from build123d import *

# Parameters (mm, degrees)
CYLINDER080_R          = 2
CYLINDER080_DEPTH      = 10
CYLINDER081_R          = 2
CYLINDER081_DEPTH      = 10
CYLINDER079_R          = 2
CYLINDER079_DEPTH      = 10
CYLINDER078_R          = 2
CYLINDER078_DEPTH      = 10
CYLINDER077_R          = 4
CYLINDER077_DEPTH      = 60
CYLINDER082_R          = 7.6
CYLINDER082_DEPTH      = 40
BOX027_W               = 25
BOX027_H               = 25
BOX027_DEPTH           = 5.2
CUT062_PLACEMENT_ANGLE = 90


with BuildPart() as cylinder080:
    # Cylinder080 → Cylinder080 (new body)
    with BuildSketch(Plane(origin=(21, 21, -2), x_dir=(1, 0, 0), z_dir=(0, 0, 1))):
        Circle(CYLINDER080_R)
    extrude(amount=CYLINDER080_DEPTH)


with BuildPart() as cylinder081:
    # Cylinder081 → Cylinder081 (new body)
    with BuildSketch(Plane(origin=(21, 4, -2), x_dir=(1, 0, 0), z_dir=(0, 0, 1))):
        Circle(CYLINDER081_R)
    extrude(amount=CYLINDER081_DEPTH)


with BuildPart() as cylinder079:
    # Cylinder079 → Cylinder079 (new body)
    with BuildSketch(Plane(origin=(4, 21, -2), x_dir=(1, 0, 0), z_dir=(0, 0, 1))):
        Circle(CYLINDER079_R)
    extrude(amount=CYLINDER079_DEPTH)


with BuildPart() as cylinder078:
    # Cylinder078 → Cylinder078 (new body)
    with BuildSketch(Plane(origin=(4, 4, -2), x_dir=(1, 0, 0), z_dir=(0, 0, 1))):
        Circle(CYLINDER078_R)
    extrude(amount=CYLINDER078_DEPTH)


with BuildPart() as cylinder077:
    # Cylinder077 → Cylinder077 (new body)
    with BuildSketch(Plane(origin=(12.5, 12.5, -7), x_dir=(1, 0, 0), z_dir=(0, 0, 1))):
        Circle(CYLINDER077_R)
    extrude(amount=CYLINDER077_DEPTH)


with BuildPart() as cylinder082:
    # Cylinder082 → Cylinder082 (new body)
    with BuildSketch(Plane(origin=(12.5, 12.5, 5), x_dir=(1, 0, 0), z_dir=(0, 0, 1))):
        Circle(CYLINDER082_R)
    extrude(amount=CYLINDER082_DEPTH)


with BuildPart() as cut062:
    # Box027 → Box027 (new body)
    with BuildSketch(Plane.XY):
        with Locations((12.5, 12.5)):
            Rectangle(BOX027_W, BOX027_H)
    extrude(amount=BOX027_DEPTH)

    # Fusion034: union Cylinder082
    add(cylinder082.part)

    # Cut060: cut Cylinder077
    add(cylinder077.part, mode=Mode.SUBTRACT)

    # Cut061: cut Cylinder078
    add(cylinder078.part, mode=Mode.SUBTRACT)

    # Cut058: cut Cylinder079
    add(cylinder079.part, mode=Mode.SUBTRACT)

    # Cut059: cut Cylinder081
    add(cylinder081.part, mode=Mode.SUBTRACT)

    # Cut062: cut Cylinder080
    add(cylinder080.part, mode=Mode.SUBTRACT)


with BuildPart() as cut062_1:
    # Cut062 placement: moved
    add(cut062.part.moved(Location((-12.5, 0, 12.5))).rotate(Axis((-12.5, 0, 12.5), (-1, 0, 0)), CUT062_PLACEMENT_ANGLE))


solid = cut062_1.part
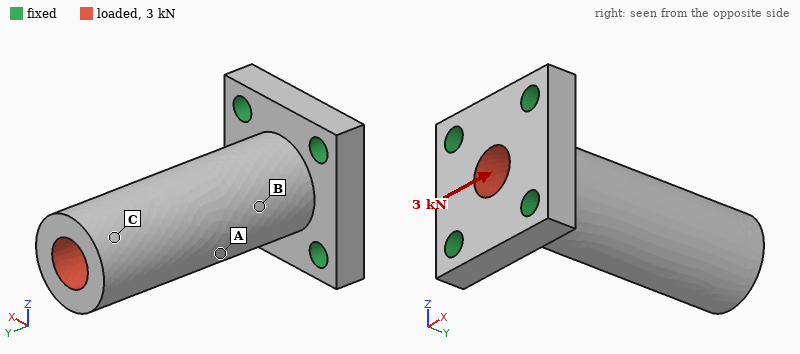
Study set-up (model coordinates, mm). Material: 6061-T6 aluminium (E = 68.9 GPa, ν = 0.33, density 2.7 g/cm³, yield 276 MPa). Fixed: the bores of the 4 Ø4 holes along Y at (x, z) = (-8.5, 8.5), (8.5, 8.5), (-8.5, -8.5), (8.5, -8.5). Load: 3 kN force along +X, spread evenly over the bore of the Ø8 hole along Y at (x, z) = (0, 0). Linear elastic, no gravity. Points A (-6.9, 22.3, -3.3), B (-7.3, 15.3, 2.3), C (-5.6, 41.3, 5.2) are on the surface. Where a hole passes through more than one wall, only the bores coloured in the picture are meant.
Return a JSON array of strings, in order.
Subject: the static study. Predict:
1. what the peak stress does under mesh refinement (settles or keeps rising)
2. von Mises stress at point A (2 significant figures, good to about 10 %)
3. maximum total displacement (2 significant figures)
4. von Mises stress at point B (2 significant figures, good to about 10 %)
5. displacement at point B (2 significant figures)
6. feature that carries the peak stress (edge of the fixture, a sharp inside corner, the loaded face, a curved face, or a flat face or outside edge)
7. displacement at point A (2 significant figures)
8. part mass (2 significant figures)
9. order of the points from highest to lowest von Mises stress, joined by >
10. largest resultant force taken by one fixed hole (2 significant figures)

["keeps rising", "50 MPa", "0.24 mm", "87 MPa", "0.059 mm", "edge of the fixture", "0.097 mm", "21 g", "B > A > C", "2.2 kN"]
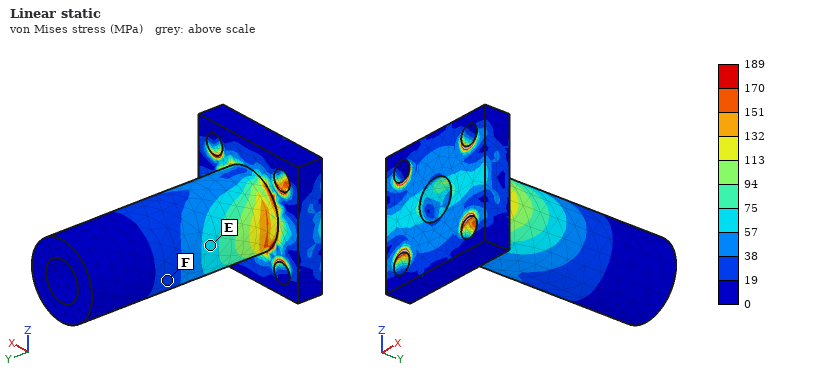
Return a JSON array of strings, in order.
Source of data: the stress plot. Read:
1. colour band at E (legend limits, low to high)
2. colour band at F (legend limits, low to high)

["57 to 75 MPa", "19 to 38 MPa"]
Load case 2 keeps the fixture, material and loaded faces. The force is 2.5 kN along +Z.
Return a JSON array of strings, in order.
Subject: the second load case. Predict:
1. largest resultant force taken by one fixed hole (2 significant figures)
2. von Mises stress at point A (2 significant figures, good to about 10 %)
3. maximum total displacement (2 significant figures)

["1.8 kN", "31 MPa", "0.20 mm"]
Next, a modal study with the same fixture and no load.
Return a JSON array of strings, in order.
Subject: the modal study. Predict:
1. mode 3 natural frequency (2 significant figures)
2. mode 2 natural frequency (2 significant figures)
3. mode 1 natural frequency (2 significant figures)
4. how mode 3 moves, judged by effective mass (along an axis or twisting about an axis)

["18 kHz", "5500 Hz", "5400 Hz", "twisting about Y"]
